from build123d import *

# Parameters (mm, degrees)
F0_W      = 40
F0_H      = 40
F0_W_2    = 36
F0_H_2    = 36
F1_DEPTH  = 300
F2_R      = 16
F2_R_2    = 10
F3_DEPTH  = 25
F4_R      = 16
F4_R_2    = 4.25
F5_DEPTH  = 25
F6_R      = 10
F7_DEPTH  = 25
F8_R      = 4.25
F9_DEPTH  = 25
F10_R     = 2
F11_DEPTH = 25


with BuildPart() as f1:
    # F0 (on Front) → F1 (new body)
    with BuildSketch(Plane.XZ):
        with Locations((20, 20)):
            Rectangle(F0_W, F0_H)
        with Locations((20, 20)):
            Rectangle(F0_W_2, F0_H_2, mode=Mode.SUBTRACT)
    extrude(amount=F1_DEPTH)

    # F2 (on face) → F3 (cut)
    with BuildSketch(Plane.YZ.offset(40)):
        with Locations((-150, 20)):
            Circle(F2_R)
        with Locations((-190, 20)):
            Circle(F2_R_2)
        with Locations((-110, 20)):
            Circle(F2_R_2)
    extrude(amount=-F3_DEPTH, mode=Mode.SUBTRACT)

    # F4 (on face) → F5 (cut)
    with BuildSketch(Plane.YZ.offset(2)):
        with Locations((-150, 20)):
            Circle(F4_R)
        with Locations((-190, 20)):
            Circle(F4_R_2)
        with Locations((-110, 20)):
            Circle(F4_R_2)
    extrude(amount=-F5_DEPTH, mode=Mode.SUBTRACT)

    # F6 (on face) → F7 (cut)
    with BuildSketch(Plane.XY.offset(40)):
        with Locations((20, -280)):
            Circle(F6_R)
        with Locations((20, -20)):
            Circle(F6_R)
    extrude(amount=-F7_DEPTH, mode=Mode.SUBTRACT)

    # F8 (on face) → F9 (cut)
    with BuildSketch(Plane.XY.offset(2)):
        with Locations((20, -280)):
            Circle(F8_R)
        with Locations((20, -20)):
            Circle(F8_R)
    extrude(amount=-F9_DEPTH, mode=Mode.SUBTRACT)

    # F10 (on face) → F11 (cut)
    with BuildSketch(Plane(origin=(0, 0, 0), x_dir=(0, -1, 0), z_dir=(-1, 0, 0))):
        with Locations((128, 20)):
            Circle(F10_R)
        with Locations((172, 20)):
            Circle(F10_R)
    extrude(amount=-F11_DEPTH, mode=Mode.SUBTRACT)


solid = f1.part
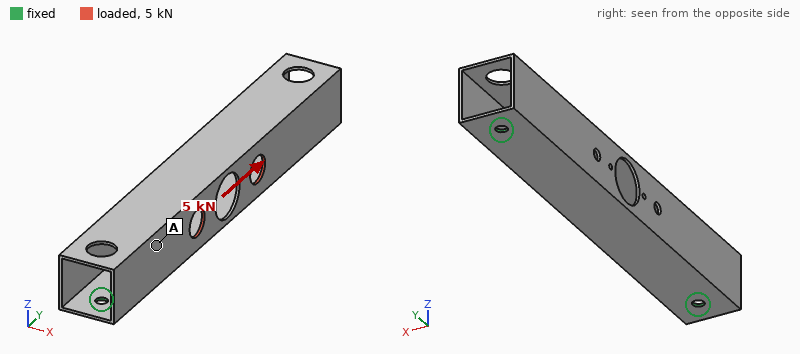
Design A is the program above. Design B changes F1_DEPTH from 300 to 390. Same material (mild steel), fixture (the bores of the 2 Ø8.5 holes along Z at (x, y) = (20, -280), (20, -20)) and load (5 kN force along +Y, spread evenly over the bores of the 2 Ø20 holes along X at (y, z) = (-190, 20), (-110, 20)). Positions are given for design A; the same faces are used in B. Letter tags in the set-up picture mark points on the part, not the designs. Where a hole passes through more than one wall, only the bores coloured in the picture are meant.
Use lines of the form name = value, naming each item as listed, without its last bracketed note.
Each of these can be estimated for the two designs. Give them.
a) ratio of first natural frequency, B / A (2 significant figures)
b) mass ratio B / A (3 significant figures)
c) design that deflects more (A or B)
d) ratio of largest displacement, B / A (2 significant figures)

ratio of first natural frequency, B / A = 0.93
mass ratio B / A = 1.32
design that deflects more = B
ratio of largest displacement, B / A = 1.3
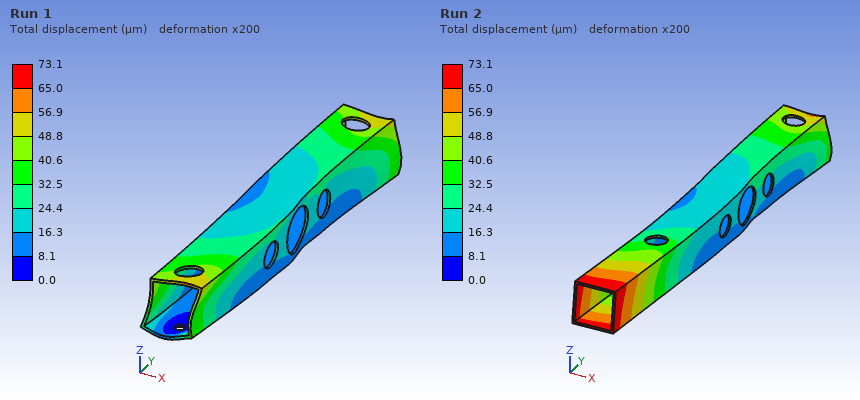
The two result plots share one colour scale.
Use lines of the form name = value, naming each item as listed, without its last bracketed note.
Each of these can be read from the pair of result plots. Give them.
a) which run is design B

which run is design B = Run 2
